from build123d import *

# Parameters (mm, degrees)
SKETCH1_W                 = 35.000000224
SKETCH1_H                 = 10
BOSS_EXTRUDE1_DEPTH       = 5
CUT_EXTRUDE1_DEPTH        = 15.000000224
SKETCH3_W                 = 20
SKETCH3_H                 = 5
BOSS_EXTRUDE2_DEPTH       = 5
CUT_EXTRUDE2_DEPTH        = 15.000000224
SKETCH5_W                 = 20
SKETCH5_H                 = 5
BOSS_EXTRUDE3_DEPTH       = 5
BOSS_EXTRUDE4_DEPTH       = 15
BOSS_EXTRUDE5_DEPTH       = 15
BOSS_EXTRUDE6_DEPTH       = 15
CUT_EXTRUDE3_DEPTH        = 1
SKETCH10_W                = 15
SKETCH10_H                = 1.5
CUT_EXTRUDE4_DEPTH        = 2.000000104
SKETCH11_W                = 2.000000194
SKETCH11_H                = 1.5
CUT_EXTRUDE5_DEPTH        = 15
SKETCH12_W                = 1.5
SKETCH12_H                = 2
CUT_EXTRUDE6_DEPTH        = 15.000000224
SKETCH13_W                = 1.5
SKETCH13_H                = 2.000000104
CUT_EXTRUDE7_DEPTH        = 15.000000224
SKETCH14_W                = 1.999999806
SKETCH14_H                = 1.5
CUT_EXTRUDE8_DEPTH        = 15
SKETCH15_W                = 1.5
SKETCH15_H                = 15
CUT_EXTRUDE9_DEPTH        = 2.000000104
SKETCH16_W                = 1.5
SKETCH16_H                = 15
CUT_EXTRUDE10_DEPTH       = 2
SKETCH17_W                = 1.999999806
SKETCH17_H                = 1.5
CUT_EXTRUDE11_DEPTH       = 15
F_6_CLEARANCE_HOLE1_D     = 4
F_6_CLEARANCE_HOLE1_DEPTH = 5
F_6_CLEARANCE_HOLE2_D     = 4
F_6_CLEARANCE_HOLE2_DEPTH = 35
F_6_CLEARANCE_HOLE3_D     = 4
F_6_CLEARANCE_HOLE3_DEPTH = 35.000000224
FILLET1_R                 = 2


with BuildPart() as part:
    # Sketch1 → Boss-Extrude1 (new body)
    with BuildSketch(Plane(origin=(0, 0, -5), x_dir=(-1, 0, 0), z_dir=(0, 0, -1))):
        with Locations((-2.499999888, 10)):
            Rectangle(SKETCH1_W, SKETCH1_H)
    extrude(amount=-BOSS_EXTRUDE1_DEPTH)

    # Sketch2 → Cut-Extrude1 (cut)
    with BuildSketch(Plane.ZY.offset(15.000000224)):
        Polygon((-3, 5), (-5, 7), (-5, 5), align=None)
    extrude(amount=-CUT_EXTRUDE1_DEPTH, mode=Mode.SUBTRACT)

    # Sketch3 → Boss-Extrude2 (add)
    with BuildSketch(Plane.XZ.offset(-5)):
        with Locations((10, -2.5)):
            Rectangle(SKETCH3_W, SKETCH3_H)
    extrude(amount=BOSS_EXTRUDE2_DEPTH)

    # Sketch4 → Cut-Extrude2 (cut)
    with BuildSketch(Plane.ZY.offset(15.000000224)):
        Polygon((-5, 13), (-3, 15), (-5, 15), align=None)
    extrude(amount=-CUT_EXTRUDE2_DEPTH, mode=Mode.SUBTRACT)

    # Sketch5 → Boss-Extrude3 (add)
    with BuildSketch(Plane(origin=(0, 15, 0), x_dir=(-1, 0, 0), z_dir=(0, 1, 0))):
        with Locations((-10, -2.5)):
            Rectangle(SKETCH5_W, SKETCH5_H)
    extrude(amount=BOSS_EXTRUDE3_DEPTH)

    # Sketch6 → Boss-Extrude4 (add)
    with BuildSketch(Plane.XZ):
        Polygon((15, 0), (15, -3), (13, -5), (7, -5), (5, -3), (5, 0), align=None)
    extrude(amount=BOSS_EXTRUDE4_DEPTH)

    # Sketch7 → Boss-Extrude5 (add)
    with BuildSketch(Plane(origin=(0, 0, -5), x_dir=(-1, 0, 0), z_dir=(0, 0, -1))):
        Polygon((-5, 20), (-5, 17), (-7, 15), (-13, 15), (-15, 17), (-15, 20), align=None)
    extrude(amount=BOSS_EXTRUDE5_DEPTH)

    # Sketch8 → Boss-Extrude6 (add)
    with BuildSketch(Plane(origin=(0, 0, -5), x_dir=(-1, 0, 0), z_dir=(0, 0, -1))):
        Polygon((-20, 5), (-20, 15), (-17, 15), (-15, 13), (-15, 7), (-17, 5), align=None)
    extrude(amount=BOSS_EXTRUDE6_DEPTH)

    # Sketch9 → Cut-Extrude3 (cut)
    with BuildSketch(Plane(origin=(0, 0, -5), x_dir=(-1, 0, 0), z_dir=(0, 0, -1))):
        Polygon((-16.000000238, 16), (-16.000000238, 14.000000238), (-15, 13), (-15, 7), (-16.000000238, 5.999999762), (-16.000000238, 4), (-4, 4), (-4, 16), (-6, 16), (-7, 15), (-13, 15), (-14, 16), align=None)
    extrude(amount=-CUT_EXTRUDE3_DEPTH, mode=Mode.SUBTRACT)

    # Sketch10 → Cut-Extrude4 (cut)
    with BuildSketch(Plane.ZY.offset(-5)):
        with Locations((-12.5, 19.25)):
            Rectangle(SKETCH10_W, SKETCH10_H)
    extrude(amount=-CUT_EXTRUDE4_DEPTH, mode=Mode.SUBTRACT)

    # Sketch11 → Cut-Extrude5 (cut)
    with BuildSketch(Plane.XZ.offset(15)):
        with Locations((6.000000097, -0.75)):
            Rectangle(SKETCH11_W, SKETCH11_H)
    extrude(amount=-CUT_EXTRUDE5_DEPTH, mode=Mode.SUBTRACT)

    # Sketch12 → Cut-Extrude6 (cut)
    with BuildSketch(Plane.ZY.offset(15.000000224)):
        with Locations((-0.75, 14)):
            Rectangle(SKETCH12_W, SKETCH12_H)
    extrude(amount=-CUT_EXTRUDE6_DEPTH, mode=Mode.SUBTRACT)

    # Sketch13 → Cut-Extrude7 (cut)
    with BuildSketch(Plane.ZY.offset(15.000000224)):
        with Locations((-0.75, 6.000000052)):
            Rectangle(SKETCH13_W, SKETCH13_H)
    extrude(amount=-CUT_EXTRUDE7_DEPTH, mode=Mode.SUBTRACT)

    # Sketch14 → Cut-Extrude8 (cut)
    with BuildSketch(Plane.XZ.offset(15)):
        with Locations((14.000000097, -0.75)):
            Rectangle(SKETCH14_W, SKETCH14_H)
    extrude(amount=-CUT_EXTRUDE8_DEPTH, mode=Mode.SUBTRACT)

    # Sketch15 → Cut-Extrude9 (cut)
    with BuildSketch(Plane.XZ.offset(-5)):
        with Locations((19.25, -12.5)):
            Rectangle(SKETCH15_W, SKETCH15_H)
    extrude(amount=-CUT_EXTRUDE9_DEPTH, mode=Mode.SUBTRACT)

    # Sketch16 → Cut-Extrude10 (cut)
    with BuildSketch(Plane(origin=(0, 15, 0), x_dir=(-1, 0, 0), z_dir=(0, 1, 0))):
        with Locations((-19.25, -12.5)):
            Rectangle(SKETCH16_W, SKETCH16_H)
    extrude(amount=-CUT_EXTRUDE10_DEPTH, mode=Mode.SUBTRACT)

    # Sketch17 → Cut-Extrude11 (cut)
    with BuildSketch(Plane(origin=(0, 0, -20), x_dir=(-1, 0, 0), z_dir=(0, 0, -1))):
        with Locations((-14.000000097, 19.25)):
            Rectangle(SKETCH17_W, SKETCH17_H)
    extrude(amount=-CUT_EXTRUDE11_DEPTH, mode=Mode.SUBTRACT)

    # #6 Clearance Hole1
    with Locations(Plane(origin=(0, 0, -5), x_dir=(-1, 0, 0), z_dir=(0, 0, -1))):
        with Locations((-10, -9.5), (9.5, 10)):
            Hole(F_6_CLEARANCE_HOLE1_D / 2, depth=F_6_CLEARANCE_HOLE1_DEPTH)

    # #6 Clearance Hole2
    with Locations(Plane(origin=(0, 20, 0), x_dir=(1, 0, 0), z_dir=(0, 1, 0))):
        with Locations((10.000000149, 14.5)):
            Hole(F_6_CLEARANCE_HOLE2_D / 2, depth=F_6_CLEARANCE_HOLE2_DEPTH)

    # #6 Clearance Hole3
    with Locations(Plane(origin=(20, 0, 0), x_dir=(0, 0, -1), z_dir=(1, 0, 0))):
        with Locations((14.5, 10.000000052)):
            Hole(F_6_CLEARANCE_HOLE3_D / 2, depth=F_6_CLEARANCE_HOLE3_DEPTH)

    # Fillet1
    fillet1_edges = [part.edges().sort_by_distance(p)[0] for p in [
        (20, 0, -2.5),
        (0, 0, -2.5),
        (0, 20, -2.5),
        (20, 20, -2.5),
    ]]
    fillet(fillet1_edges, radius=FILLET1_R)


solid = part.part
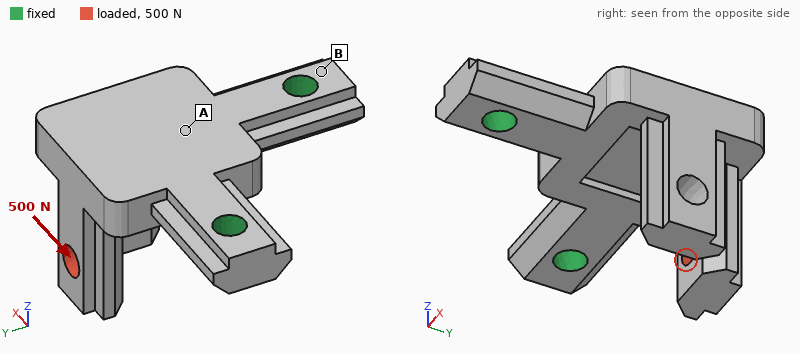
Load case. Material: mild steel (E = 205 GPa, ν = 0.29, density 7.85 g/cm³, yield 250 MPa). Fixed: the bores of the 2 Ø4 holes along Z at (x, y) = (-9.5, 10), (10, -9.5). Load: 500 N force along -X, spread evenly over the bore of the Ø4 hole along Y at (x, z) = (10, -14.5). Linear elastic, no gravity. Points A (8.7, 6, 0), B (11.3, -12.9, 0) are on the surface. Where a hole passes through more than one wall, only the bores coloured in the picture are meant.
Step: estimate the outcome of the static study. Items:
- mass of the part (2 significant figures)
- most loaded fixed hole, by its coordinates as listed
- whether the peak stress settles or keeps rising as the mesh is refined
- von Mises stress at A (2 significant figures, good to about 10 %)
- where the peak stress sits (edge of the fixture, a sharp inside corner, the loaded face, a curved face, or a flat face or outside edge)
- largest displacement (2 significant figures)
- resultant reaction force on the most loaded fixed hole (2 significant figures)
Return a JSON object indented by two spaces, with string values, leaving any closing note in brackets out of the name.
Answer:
{
  "mass of the part": "31 g",
  "most loaded fixed hole, by its coordinates as listed": "(-9.5, 10)",
  "whether the peak stress settles or keeps rising as the mesh is refined": "keeps rising",
  "von Mises stress at A": "56 MPa",
  "where the peak stress sits": "a sharp inside corner",
  "largest displacement": "80 µm",
  "resultant reaction force on the most loaded fixed hole": "590 N"
}
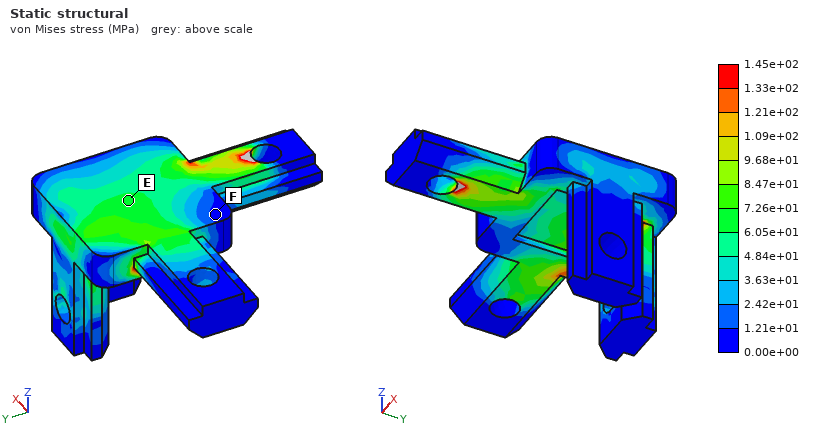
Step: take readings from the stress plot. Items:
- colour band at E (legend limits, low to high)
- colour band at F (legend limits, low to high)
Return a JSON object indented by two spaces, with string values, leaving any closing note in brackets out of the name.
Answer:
{
  "colour band at E": "6.05e+01 to 7.26e+01 MPa",
  "colour band at F": "0.00e+00 to 1.21e+01 MPa"
}
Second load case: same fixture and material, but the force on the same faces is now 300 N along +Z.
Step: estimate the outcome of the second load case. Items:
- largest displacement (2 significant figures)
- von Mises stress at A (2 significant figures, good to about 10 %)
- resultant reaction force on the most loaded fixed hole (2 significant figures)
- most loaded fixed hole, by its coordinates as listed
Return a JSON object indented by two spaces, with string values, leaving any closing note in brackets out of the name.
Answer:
{
  "largest displacement": "52 µm",
  "von Mises stress at A": "32 MPa",
  "resultant reaction force on the most loaded fixed hole": "220 N",
  "most loaded fixed hole, by its coordinates as listed": "(-9.5, 10)"
}
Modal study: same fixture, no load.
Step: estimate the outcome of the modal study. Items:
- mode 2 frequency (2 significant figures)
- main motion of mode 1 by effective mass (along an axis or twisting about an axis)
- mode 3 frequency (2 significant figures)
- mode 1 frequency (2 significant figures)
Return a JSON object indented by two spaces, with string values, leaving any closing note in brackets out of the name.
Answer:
{
  "mode 2 frequency": "7500 Hz",
  "main motion of mode 1 by effective mass": "along Z",
  "mode 3 frequency": "10 kHz",
  "mode 1 frequency": "3500 Hz"
}
